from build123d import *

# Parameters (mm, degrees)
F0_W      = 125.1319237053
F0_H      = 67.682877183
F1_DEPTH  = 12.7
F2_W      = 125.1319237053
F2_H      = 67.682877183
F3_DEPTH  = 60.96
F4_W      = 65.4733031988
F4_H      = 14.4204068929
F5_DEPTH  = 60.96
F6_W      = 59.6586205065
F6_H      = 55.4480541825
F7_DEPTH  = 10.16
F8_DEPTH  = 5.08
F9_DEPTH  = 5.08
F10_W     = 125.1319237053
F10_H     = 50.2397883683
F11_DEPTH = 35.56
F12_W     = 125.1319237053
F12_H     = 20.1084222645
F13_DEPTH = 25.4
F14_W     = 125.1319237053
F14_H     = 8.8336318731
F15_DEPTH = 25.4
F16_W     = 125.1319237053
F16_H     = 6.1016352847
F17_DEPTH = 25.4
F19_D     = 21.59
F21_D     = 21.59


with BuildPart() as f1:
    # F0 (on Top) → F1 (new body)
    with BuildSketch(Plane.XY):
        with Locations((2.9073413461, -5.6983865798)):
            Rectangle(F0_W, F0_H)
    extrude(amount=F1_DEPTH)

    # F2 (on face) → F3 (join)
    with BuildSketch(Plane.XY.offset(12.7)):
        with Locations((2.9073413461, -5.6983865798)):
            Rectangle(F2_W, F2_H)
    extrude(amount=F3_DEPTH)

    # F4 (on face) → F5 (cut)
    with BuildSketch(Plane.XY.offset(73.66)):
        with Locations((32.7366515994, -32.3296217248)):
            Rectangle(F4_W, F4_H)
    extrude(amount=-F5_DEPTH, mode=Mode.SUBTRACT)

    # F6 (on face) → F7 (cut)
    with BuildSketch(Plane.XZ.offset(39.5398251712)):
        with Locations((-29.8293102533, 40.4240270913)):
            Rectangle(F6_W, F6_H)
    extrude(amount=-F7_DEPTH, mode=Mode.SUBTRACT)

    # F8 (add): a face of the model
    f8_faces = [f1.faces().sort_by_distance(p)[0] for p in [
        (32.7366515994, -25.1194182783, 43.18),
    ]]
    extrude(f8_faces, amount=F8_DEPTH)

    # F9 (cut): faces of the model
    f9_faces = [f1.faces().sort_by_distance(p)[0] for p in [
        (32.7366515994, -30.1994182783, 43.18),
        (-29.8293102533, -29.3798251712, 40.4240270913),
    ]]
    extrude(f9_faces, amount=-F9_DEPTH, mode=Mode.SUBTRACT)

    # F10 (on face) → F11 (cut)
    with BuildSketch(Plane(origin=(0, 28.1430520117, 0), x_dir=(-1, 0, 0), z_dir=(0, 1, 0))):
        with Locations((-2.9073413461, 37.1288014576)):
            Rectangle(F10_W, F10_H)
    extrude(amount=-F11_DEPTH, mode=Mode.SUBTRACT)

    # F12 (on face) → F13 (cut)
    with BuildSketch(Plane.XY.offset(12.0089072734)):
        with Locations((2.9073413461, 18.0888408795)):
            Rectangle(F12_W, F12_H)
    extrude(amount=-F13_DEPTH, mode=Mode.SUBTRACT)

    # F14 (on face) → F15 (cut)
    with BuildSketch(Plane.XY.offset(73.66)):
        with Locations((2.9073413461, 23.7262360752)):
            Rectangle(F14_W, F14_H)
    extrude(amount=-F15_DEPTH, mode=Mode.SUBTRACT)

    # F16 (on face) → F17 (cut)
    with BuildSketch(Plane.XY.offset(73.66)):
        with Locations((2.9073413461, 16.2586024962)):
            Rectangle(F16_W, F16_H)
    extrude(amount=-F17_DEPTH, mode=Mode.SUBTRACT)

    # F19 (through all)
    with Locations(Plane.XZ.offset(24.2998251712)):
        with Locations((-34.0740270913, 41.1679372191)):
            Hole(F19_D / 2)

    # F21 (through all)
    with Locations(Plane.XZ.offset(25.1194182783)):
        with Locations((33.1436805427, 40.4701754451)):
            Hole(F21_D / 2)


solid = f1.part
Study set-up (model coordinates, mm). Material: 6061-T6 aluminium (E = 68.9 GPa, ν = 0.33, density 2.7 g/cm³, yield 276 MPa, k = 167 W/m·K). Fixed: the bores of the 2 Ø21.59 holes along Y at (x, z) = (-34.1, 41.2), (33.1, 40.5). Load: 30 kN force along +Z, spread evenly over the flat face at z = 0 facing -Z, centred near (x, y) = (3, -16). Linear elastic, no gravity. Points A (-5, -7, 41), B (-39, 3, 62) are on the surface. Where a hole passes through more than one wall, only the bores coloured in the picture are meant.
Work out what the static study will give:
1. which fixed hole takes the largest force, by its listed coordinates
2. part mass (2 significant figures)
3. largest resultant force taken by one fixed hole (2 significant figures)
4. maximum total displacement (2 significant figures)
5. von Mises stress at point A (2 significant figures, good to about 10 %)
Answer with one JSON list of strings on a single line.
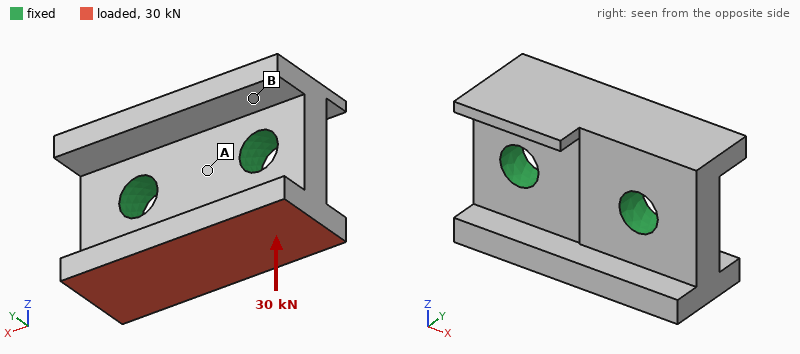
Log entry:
["(33.1, 40.5)", "620 g", "16 kN", "23 µm", "5.8 MPa"]
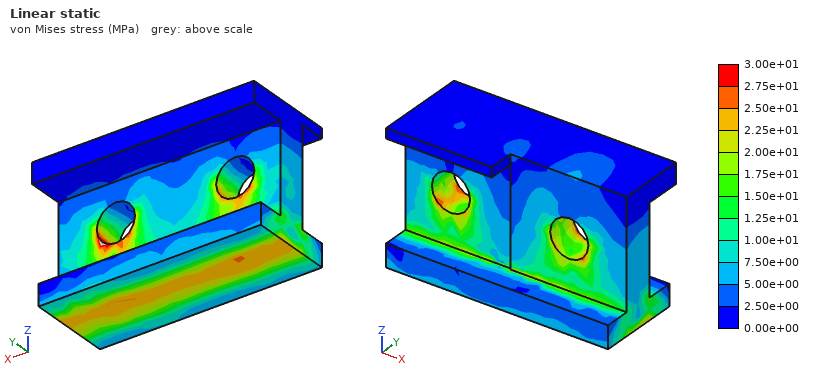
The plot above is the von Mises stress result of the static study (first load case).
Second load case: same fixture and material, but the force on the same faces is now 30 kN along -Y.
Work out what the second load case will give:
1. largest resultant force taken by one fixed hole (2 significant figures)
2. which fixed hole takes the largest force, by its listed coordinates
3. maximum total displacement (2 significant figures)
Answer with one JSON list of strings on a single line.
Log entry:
["16 kN", "(33.1, 40.5)", "0.19 mm"]
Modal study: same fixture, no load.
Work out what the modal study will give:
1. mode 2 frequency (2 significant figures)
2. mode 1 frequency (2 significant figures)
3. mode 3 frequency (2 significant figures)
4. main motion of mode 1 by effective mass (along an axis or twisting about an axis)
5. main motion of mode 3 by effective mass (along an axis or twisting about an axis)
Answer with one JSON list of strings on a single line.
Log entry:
["6600 Hz", "5500 Hz", "7400 Hz", "along Y", "along Y"]
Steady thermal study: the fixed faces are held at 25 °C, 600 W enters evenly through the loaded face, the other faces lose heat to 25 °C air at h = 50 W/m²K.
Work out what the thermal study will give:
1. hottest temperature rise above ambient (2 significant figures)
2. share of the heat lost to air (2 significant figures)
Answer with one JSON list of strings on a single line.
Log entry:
["57 K", "5.2 %"]
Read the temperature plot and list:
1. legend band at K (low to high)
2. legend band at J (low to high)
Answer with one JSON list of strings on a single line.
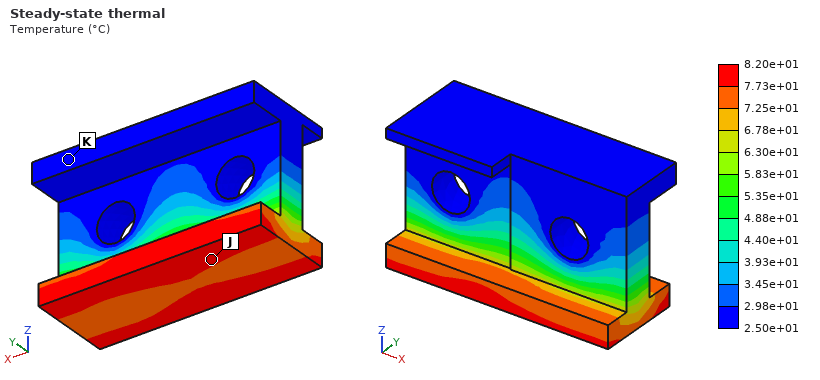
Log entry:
["2.50e+01 to 2.98e+01 °C", "7.73e+01 to 8.20e+01 °C"]
